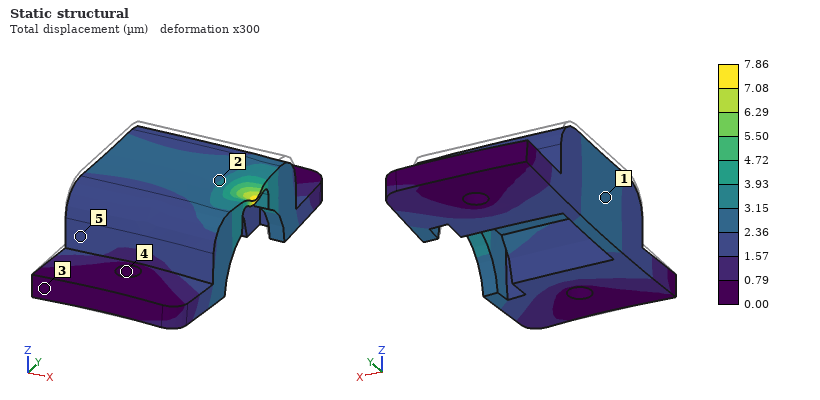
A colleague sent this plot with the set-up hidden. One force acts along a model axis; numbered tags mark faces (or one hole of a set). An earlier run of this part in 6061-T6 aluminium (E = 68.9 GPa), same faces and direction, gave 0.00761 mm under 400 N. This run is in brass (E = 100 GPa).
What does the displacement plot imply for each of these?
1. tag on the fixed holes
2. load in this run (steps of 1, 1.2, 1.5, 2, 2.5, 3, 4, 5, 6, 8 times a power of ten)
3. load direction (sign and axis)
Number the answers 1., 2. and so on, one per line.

1. 4
2. 600 N
3. -Z
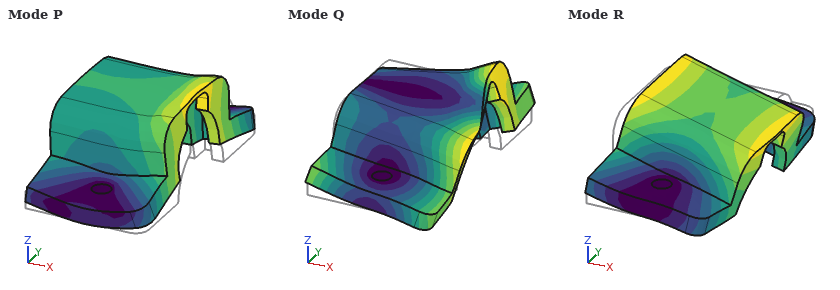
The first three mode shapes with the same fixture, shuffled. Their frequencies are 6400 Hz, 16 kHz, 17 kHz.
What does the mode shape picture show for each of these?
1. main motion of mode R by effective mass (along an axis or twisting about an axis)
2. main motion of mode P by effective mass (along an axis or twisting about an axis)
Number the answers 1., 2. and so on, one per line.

1. along X
2. along Z
